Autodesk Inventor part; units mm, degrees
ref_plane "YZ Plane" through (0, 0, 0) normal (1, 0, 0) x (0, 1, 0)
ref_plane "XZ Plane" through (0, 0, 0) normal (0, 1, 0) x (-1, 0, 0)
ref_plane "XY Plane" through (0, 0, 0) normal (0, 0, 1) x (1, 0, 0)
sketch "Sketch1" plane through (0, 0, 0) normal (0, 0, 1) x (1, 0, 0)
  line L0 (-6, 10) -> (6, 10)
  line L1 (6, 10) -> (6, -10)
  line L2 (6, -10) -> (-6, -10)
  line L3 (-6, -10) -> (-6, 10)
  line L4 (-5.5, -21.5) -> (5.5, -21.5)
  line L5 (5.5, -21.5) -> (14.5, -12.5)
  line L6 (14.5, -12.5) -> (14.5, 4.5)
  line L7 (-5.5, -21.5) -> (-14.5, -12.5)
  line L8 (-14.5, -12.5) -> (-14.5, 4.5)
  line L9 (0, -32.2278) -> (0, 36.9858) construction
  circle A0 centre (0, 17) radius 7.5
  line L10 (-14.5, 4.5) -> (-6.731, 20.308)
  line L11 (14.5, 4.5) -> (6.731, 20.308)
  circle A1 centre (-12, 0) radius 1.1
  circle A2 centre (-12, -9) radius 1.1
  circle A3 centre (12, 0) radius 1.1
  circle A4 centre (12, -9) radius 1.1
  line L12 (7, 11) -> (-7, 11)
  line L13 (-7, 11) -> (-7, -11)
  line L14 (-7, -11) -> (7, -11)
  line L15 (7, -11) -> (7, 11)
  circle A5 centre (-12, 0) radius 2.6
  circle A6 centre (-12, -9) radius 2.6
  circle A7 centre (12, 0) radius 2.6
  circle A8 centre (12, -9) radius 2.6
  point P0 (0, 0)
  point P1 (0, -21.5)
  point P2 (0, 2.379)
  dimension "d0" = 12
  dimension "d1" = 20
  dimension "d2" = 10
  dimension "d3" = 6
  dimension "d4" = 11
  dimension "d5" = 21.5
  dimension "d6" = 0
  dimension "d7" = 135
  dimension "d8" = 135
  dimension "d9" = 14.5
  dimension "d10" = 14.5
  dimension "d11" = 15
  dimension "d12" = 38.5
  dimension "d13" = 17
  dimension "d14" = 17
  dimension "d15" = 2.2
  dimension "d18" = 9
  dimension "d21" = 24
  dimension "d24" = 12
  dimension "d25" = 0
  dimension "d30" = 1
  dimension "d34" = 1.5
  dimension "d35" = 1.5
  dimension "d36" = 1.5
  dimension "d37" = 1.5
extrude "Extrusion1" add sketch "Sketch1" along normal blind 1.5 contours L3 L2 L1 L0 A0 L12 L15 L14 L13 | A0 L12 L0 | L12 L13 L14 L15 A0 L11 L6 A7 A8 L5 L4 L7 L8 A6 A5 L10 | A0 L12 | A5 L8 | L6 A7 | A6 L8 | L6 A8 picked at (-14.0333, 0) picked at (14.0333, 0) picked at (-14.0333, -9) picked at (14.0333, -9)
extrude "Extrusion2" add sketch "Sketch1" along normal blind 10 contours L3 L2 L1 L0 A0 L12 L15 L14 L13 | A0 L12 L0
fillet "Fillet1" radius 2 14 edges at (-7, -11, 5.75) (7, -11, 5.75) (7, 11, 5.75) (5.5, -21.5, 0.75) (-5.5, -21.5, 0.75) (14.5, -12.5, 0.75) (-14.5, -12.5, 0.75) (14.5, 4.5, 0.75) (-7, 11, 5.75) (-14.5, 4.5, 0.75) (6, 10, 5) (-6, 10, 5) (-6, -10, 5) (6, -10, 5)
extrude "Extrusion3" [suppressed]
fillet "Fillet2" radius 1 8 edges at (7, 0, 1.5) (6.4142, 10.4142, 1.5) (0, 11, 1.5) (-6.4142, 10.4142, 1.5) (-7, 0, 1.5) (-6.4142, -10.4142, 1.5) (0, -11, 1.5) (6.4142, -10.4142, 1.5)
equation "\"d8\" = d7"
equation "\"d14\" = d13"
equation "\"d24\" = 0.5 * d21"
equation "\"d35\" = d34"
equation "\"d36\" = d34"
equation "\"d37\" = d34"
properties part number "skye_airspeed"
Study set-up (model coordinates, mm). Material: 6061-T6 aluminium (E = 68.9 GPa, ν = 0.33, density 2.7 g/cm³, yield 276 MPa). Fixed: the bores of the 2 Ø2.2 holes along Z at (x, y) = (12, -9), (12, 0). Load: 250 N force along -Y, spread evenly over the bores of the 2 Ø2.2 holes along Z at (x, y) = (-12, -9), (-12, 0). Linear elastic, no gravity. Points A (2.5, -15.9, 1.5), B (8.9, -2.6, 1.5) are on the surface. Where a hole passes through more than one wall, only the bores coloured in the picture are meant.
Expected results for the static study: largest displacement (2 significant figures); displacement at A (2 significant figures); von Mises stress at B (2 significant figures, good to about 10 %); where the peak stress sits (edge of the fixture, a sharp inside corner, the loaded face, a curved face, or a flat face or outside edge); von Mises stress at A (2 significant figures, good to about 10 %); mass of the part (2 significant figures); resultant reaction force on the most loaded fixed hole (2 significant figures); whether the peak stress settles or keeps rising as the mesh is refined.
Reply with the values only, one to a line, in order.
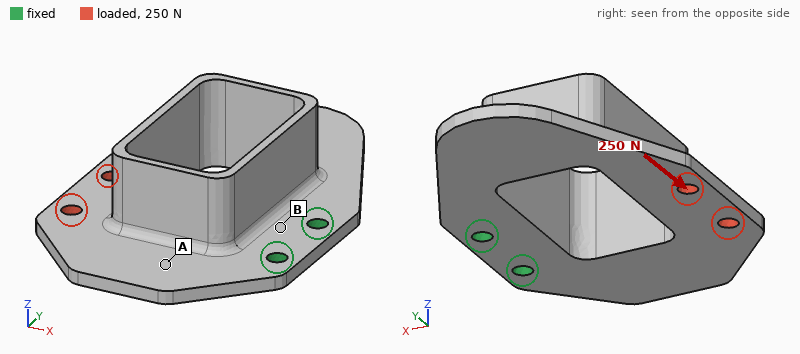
0.12 mm
0.045 mm
80 MPa
edge of the fixture
31 MPa
4.8 g
500 N
keeps rising
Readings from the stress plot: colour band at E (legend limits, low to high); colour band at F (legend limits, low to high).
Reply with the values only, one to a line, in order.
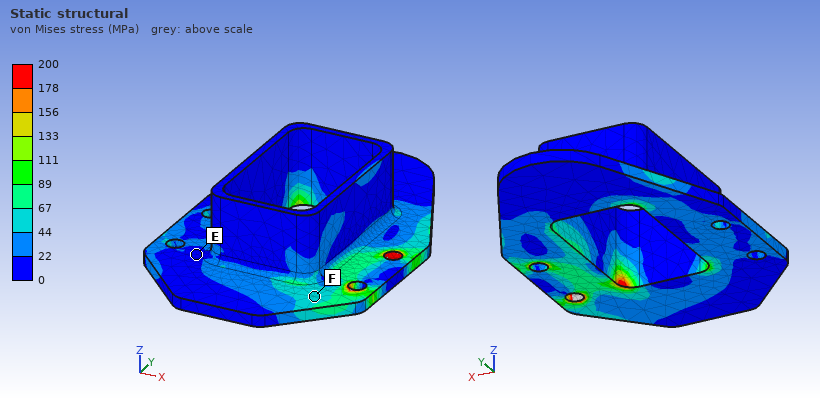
0 to 22 MPa
44 to 67 MPa
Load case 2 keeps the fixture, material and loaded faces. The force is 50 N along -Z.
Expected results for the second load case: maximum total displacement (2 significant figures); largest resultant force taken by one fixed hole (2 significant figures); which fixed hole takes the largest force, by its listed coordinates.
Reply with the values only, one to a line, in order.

0.43 mm
45 N
(12, 0)
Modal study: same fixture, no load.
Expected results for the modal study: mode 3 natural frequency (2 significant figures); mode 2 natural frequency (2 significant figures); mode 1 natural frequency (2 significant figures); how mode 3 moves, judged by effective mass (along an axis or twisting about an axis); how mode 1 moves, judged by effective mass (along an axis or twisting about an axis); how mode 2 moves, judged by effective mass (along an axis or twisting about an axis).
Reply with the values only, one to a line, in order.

5400 Hz
2600 Hz
1500 Hz
along Y
along Z
twisting about X
